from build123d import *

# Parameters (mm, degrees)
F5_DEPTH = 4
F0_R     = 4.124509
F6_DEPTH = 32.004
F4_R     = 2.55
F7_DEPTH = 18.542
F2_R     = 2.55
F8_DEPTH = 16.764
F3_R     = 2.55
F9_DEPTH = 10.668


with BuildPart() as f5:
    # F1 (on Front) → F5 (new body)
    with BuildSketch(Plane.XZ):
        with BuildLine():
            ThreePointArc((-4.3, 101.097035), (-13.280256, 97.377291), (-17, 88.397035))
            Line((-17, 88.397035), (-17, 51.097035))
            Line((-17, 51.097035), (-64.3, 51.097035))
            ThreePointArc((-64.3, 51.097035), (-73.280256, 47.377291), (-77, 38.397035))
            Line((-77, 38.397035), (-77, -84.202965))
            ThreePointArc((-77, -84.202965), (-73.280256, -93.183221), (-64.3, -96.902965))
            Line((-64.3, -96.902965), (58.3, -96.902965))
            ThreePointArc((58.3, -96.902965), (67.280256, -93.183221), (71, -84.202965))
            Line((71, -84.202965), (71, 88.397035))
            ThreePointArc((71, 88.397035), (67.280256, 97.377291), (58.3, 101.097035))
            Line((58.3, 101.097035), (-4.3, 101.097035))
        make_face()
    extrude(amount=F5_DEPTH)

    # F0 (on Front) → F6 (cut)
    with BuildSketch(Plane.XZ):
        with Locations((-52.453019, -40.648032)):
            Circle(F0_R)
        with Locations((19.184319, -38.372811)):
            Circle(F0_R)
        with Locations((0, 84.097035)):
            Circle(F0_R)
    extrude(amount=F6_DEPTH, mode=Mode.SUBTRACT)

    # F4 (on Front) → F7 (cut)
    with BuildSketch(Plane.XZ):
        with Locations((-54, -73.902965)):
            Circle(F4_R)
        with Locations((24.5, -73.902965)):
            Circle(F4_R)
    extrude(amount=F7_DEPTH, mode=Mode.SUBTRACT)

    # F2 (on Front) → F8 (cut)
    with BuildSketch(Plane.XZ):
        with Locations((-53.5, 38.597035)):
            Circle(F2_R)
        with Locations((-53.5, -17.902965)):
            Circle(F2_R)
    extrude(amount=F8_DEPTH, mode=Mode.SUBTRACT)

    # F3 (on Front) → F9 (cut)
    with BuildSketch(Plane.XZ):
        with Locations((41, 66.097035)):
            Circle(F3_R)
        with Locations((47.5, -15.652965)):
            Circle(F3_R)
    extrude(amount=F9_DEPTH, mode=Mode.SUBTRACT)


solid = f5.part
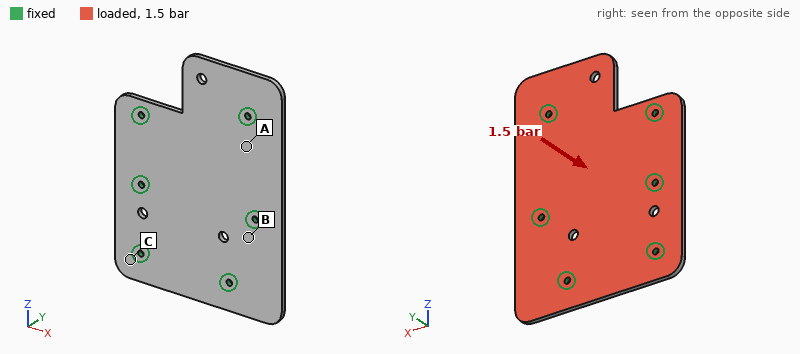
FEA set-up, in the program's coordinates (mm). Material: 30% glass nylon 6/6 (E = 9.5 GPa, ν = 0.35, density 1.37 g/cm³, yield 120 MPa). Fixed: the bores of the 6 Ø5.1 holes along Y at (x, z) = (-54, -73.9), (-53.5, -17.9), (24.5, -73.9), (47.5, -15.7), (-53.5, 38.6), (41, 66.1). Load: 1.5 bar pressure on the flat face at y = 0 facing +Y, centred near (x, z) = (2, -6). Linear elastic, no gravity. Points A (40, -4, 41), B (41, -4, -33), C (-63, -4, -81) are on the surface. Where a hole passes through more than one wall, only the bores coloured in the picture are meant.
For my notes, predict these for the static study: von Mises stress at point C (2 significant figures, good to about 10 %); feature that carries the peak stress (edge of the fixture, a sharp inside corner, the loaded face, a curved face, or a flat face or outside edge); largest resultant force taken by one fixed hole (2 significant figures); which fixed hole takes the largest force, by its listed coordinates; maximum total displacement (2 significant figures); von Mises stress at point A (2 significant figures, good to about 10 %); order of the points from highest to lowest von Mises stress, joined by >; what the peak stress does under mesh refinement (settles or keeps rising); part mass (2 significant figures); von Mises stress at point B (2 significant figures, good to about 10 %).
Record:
6.8 MPa
edge of the fixture
900 N
(41, 66.1)
2.5 mm
17 MPa
B > A > C
keeps rising
140 g
23 MPa
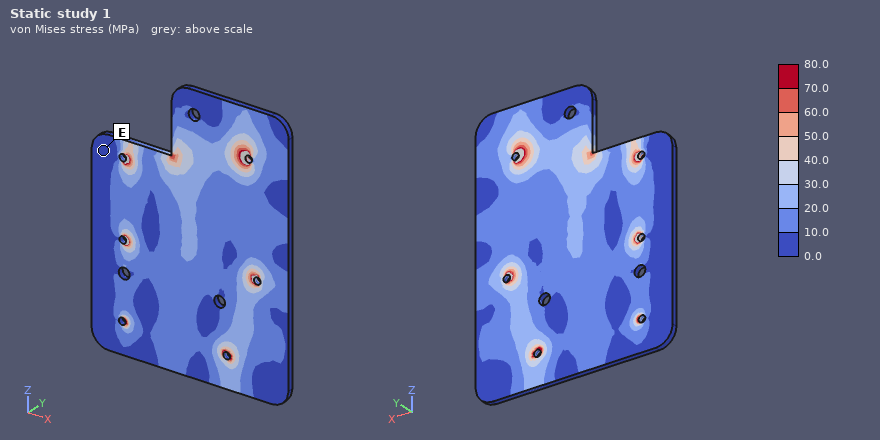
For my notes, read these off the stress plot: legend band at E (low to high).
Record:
0.0 to 10.0 MPa
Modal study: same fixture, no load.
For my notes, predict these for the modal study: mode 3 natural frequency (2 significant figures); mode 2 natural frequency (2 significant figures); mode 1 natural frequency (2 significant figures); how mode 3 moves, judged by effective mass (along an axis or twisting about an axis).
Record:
1000 Hz
920 Hz
700 Hz
along Y
